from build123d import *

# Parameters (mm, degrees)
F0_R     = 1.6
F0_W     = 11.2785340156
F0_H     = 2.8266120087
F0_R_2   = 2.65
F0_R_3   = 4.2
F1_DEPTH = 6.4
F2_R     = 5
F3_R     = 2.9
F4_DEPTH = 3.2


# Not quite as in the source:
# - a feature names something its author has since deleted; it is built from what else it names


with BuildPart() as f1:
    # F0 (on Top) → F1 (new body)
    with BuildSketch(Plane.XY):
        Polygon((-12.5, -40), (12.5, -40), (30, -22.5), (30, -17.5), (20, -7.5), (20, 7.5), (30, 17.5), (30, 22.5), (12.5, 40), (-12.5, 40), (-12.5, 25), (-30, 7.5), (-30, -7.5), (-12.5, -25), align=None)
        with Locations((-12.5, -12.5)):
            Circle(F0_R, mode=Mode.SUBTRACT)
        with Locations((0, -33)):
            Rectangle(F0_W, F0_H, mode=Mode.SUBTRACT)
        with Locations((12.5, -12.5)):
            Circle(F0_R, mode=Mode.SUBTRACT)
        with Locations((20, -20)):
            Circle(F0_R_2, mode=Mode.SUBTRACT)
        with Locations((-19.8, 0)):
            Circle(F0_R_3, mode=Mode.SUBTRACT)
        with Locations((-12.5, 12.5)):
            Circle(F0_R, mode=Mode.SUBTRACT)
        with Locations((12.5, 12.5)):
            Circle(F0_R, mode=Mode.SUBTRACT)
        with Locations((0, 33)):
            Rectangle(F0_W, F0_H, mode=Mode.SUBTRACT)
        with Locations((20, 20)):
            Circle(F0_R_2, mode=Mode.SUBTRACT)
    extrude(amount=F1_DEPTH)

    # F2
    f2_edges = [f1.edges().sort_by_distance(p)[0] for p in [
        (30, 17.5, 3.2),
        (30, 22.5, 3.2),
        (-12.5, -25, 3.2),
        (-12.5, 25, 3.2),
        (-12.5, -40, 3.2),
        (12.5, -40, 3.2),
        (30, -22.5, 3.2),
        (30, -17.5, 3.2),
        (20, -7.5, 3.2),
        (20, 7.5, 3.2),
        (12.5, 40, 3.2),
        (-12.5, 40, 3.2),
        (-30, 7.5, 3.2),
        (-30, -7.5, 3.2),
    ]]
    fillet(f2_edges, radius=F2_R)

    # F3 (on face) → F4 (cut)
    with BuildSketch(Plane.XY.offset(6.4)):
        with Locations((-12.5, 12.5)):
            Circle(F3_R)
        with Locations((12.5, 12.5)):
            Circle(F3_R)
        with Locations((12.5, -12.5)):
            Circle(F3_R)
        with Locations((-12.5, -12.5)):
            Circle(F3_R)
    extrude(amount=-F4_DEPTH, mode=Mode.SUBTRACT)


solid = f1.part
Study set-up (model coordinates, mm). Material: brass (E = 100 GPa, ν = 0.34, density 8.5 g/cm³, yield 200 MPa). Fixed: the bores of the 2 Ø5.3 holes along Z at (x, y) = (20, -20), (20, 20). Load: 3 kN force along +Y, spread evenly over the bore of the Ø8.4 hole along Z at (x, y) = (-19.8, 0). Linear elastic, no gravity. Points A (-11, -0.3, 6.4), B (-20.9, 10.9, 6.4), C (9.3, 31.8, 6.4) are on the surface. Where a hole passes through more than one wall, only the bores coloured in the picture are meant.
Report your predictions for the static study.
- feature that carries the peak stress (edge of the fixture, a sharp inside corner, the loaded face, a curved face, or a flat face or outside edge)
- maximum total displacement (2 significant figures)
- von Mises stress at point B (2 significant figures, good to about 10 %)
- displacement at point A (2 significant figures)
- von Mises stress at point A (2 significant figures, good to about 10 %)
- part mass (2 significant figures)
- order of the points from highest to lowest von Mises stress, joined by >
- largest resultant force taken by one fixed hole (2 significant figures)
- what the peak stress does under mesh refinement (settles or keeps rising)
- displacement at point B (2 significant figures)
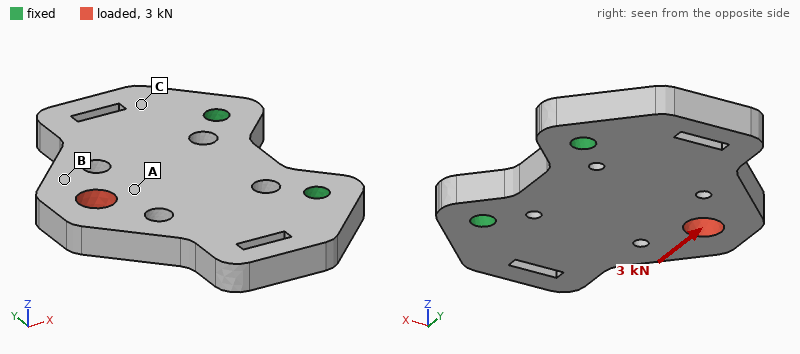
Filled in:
edge of the fixture
23 µm
21 MPa
14 µm
30 MPa
170 g
A > B > C
3.1 kN
keeps rising
20 µm
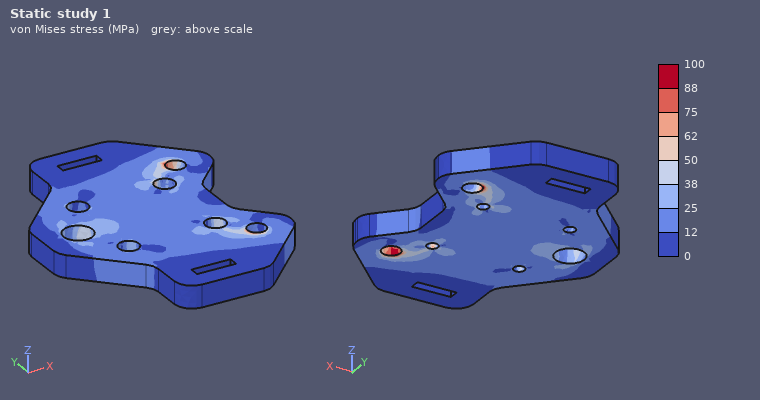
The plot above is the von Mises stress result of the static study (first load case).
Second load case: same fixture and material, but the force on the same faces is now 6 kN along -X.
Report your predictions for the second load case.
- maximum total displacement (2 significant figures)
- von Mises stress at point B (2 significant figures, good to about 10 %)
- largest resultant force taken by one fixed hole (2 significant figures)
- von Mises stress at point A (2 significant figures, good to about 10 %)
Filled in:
19 µm
19 MPa
3.2 kN
34 MPa
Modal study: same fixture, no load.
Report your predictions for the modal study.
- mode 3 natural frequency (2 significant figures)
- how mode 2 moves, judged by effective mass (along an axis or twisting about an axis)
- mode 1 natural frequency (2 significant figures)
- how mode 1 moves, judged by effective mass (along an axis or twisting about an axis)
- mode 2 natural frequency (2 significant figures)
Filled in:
5200 Hz
twisting about X
1700 Hz
along Z
3500 Hz
